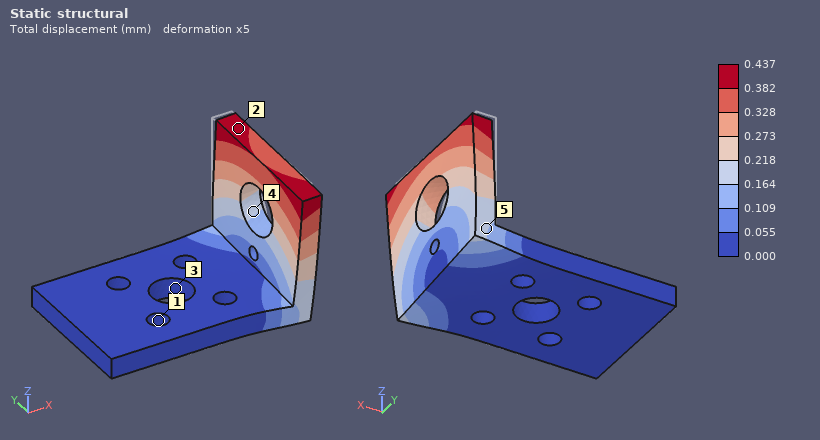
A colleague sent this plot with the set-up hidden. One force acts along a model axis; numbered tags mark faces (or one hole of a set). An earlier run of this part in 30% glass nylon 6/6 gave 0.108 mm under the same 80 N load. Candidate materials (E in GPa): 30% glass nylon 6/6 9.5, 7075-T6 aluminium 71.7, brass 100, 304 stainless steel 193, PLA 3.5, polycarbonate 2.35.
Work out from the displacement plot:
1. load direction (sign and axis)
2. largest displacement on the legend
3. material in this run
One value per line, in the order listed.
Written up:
-Y
0.437 mm
polycarbonate
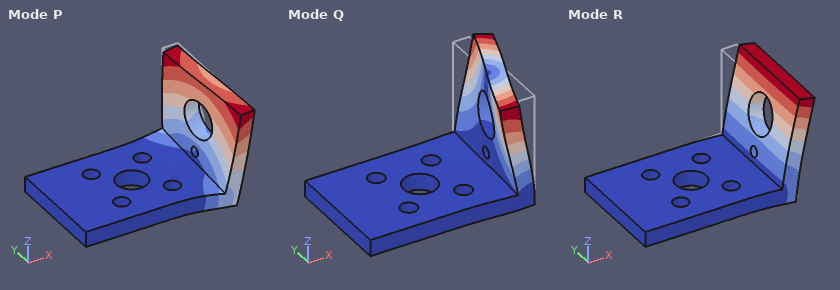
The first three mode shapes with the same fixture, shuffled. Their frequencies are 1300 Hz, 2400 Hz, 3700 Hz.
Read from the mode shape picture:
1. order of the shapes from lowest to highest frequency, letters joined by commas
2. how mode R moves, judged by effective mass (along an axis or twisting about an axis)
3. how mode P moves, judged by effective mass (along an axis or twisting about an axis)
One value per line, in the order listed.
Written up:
R, P, Q
along X
along Y
